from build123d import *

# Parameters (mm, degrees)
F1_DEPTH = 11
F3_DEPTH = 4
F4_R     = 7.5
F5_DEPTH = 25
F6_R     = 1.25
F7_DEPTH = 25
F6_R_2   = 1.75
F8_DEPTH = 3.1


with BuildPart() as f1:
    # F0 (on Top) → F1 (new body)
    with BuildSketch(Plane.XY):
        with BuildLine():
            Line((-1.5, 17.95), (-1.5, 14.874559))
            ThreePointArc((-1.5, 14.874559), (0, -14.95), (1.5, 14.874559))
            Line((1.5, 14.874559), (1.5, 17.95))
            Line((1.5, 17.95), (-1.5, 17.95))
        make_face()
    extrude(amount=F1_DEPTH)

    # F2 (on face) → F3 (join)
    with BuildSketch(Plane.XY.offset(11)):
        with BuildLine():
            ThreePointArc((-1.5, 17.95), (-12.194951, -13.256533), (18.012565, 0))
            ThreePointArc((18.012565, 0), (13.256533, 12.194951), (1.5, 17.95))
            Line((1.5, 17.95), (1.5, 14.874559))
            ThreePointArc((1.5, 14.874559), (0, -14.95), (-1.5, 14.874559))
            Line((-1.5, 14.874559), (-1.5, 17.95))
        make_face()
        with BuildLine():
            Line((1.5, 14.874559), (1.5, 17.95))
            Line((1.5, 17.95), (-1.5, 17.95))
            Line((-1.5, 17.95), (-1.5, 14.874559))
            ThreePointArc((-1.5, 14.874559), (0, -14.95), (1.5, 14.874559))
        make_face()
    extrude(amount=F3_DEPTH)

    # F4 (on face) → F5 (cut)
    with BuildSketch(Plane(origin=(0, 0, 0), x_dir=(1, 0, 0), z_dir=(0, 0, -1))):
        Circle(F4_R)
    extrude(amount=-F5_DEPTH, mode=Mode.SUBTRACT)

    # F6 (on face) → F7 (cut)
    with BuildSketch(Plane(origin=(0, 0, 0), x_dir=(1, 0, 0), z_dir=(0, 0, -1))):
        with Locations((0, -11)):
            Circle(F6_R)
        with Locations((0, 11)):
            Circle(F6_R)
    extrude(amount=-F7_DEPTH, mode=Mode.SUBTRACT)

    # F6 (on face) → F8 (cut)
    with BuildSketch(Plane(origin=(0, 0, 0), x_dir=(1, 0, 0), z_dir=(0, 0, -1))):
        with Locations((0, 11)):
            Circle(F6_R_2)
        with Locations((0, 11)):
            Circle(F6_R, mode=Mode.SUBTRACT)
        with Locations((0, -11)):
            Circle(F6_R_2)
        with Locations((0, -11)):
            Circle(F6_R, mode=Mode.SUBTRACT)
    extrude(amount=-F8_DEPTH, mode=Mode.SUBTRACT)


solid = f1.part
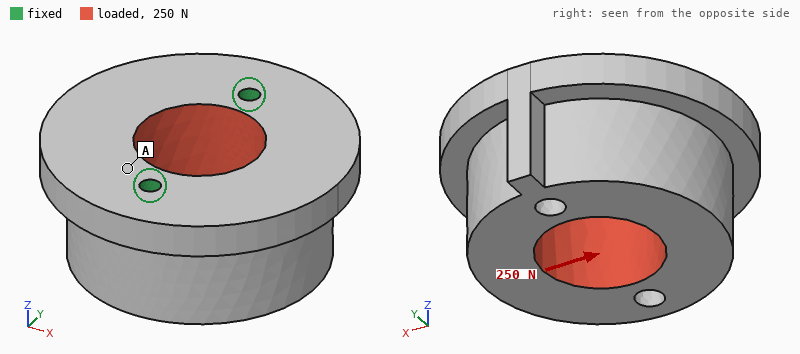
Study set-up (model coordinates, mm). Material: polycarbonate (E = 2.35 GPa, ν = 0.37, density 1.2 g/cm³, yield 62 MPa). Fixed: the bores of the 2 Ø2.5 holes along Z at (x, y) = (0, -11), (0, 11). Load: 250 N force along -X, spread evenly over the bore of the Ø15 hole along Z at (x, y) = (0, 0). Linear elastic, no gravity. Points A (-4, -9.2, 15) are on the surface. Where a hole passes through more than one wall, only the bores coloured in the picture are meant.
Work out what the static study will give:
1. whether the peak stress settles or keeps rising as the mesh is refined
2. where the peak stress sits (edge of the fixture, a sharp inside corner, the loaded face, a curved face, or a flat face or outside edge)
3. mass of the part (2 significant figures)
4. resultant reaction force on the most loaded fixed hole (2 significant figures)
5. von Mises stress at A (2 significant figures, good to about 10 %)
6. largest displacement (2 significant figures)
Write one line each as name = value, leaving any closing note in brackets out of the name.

whether the peak stress settles or keeps rising as the mesh is refined = keeps rising
where the peak stress sits = edge of the fixture
mass of the part = 11 g
resultant reaction force on the most loaded fixed hole = 130 N
von Mises stress at A = 0.55 MPa
largest displacement = 7.6 µm
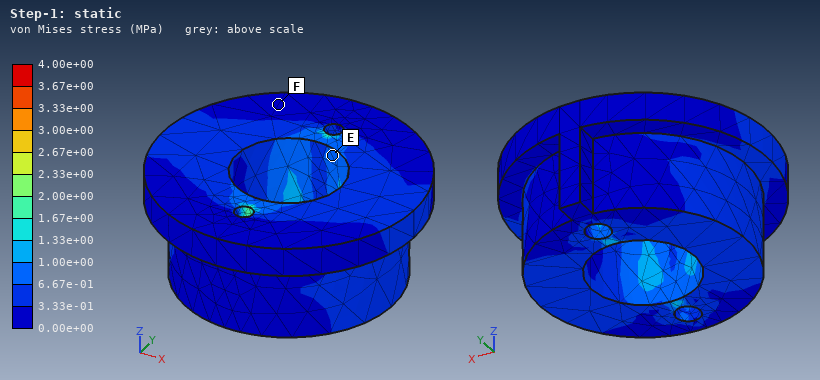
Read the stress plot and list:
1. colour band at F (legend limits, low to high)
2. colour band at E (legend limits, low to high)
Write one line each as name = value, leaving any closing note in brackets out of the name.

colour band at F = 0.00e+00 to 3.33e-01 MPa
colour band at E = 6.67e-01 to 1.00e+00 MPa
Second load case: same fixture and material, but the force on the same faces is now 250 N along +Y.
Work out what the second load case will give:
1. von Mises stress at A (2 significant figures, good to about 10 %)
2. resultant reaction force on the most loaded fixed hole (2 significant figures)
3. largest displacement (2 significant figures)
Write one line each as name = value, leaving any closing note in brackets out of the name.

von Mises stress at A = 0.91 MPa
resultant reaction force on the most loaded fixed hole = 130 N
largest displacement = 7.2 µm
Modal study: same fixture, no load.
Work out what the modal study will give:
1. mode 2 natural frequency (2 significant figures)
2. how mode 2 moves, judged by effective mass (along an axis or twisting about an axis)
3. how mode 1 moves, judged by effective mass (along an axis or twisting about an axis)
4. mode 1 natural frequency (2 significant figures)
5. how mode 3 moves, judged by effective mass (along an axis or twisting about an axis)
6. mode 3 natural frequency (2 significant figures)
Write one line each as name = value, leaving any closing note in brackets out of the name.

mode 2 natural frequency = 7100 Hz
how mode 2 moves, judged by effective mass = along Z
how mode 1 moves, judged by effective mass = twisting about Y
mode 1 natural frequency = 5900 Hz
how mode 3 moves, judged by effective mass = twisting about Z
mode 3 natural frequency = 7900 Hz
